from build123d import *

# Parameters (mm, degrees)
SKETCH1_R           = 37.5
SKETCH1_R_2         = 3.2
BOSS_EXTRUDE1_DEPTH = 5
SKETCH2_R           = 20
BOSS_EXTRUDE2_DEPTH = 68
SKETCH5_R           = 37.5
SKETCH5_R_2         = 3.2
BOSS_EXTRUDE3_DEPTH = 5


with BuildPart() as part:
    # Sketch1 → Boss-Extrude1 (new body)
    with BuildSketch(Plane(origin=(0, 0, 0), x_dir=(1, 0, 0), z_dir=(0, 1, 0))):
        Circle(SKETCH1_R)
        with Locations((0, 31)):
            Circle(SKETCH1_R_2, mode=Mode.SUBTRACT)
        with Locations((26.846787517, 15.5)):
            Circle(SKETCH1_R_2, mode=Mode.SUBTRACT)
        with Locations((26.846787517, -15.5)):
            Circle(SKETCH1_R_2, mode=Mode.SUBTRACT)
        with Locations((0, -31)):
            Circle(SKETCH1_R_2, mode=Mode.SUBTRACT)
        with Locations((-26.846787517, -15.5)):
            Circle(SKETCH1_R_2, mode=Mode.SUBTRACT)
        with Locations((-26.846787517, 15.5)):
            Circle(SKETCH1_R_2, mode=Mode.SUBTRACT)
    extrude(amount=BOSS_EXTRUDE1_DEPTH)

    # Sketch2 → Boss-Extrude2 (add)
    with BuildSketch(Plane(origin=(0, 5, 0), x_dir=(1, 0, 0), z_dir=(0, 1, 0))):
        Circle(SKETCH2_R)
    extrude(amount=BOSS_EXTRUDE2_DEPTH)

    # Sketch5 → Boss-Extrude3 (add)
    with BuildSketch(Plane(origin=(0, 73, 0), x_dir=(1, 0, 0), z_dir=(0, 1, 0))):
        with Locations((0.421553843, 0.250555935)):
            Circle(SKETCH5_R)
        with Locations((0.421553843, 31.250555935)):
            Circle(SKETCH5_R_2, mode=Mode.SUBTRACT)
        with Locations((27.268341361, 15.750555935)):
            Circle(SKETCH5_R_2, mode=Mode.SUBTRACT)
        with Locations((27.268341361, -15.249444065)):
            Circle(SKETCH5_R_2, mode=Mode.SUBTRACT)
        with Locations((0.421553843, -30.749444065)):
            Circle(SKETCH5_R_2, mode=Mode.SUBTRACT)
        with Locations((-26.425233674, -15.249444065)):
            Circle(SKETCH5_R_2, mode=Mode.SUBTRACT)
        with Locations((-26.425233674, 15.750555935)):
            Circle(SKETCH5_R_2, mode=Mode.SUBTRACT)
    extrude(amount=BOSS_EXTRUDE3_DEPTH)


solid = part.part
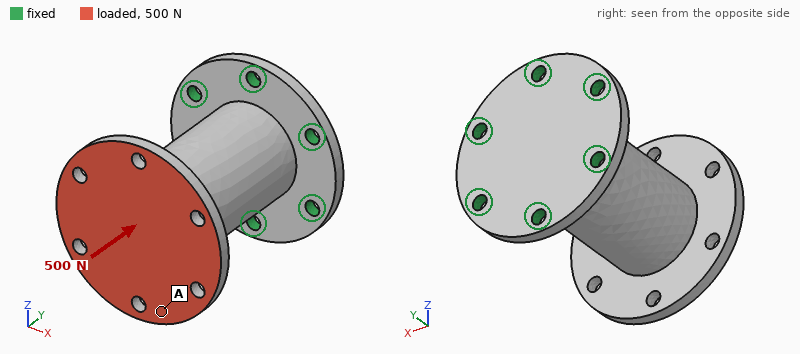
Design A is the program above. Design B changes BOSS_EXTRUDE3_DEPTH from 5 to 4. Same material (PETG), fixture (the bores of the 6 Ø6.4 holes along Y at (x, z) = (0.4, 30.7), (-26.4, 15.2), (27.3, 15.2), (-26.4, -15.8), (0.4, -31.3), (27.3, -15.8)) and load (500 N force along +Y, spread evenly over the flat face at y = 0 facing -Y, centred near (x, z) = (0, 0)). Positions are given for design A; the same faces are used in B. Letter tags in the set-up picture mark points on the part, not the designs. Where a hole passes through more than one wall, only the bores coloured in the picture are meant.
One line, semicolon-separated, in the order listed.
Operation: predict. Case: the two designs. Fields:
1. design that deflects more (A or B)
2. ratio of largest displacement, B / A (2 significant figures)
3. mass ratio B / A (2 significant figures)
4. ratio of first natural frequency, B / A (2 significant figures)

B; 1.1; 0.97; 0.85
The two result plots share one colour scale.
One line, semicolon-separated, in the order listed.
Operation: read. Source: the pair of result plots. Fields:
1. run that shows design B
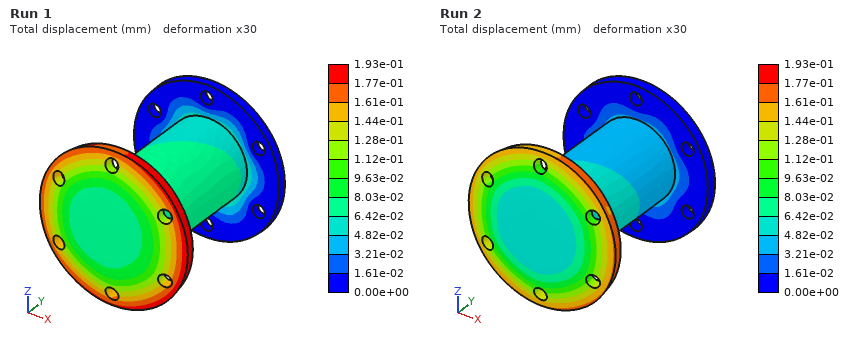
Run 1
